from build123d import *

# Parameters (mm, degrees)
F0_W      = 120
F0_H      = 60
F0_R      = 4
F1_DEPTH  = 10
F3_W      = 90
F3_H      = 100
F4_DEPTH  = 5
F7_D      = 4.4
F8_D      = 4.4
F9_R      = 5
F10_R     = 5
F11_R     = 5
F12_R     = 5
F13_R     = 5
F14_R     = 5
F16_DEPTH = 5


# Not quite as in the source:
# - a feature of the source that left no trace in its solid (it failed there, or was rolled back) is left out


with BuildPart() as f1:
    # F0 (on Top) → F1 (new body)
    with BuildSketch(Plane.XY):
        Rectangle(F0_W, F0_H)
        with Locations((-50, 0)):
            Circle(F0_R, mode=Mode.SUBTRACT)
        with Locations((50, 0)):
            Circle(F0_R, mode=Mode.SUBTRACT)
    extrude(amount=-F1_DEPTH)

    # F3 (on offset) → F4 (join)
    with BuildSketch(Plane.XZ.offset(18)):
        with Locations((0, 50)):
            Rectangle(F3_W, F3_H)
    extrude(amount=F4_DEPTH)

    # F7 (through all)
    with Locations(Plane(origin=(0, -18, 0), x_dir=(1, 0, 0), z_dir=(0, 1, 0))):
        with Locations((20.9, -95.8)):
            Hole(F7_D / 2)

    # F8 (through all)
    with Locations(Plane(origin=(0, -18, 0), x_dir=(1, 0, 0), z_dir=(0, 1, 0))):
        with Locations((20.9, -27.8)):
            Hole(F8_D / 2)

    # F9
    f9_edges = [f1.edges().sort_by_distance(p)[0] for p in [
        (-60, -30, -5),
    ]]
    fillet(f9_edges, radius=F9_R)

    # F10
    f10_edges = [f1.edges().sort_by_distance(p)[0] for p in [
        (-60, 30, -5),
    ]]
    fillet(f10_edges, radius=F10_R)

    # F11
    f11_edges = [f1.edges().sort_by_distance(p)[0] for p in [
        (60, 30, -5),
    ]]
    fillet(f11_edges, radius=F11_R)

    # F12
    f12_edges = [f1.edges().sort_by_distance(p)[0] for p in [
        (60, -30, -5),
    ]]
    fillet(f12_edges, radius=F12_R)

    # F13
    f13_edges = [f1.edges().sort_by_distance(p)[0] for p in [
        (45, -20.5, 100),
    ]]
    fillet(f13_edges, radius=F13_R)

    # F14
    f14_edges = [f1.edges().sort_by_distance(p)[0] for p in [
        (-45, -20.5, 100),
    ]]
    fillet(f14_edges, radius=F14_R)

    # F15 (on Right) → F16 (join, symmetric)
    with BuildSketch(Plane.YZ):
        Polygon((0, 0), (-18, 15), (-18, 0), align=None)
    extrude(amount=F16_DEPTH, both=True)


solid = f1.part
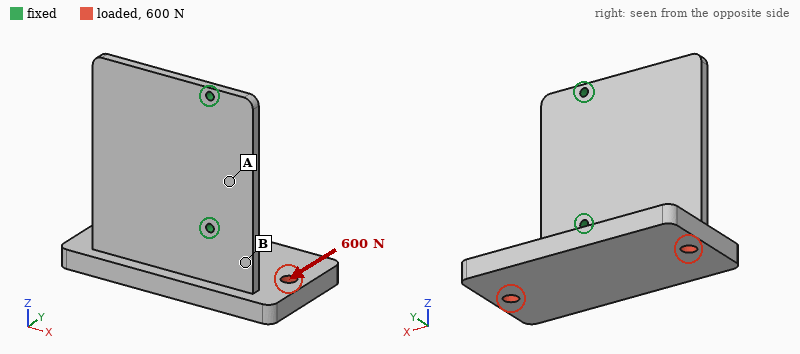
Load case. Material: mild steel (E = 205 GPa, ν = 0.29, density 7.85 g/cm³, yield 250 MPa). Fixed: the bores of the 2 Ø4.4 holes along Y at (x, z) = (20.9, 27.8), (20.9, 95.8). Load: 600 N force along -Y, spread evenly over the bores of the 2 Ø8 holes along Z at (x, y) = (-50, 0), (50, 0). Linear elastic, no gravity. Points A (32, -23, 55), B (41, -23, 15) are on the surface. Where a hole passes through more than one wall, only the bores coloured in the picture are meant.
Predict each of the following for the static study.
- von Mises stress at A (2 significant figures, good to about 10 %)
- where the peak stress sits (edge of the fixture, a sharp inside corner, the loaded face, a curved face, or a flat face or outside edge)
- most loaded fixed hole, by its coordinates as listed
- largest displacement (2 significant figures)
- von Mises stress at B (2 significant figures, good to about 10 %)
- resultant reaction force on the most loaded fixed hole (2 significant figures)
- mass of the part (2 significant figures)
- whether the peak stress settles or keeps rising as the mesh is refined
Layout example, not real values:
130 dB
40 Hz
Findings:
11 MPa
edge of the fixture
(20.9, 27.8)
0.25 mm
42 MPa
740 N
920 g
keeps rising
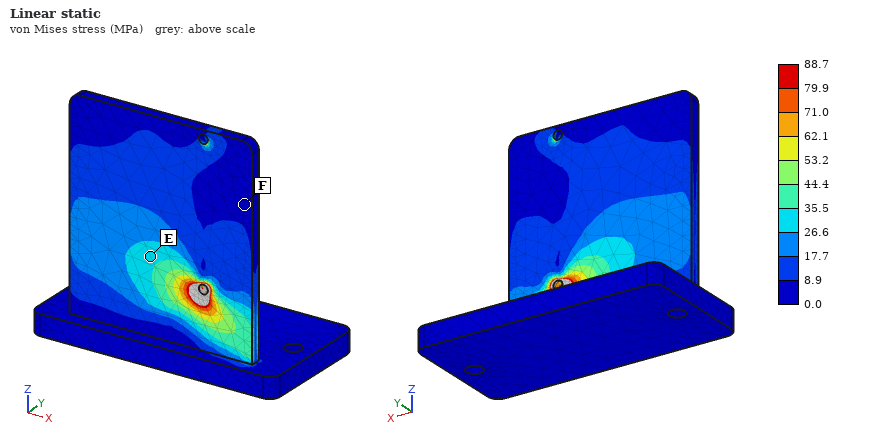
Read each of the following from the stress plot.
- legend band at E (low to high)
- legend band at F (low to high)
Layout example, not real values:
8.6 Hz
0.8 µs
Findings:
26.6 to 35.5 MPa
0.0 to 8.9 MPa
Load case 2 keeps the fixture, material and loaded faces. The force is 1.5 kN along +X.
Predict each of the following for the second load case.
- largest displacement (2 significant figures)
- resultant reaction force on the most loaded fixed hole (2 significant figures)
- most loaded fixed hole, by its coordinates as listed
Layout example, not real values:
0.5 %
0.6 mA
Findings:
0.35 mm
2.2 kN
(20.9, 27.8)
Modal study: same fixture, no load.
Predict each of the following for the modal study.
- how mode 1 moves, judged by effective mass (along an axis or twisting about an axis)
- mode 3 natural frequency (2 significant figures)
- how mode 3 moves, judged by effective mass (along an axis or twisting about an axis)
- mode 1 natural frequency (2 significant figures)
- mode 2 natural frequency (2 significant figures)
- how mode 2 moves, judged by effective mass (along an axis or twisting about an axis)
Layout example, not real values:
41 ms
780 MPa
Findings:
along Y
1300 Hz
along Y
350 Hz
530 Hz
along Z
